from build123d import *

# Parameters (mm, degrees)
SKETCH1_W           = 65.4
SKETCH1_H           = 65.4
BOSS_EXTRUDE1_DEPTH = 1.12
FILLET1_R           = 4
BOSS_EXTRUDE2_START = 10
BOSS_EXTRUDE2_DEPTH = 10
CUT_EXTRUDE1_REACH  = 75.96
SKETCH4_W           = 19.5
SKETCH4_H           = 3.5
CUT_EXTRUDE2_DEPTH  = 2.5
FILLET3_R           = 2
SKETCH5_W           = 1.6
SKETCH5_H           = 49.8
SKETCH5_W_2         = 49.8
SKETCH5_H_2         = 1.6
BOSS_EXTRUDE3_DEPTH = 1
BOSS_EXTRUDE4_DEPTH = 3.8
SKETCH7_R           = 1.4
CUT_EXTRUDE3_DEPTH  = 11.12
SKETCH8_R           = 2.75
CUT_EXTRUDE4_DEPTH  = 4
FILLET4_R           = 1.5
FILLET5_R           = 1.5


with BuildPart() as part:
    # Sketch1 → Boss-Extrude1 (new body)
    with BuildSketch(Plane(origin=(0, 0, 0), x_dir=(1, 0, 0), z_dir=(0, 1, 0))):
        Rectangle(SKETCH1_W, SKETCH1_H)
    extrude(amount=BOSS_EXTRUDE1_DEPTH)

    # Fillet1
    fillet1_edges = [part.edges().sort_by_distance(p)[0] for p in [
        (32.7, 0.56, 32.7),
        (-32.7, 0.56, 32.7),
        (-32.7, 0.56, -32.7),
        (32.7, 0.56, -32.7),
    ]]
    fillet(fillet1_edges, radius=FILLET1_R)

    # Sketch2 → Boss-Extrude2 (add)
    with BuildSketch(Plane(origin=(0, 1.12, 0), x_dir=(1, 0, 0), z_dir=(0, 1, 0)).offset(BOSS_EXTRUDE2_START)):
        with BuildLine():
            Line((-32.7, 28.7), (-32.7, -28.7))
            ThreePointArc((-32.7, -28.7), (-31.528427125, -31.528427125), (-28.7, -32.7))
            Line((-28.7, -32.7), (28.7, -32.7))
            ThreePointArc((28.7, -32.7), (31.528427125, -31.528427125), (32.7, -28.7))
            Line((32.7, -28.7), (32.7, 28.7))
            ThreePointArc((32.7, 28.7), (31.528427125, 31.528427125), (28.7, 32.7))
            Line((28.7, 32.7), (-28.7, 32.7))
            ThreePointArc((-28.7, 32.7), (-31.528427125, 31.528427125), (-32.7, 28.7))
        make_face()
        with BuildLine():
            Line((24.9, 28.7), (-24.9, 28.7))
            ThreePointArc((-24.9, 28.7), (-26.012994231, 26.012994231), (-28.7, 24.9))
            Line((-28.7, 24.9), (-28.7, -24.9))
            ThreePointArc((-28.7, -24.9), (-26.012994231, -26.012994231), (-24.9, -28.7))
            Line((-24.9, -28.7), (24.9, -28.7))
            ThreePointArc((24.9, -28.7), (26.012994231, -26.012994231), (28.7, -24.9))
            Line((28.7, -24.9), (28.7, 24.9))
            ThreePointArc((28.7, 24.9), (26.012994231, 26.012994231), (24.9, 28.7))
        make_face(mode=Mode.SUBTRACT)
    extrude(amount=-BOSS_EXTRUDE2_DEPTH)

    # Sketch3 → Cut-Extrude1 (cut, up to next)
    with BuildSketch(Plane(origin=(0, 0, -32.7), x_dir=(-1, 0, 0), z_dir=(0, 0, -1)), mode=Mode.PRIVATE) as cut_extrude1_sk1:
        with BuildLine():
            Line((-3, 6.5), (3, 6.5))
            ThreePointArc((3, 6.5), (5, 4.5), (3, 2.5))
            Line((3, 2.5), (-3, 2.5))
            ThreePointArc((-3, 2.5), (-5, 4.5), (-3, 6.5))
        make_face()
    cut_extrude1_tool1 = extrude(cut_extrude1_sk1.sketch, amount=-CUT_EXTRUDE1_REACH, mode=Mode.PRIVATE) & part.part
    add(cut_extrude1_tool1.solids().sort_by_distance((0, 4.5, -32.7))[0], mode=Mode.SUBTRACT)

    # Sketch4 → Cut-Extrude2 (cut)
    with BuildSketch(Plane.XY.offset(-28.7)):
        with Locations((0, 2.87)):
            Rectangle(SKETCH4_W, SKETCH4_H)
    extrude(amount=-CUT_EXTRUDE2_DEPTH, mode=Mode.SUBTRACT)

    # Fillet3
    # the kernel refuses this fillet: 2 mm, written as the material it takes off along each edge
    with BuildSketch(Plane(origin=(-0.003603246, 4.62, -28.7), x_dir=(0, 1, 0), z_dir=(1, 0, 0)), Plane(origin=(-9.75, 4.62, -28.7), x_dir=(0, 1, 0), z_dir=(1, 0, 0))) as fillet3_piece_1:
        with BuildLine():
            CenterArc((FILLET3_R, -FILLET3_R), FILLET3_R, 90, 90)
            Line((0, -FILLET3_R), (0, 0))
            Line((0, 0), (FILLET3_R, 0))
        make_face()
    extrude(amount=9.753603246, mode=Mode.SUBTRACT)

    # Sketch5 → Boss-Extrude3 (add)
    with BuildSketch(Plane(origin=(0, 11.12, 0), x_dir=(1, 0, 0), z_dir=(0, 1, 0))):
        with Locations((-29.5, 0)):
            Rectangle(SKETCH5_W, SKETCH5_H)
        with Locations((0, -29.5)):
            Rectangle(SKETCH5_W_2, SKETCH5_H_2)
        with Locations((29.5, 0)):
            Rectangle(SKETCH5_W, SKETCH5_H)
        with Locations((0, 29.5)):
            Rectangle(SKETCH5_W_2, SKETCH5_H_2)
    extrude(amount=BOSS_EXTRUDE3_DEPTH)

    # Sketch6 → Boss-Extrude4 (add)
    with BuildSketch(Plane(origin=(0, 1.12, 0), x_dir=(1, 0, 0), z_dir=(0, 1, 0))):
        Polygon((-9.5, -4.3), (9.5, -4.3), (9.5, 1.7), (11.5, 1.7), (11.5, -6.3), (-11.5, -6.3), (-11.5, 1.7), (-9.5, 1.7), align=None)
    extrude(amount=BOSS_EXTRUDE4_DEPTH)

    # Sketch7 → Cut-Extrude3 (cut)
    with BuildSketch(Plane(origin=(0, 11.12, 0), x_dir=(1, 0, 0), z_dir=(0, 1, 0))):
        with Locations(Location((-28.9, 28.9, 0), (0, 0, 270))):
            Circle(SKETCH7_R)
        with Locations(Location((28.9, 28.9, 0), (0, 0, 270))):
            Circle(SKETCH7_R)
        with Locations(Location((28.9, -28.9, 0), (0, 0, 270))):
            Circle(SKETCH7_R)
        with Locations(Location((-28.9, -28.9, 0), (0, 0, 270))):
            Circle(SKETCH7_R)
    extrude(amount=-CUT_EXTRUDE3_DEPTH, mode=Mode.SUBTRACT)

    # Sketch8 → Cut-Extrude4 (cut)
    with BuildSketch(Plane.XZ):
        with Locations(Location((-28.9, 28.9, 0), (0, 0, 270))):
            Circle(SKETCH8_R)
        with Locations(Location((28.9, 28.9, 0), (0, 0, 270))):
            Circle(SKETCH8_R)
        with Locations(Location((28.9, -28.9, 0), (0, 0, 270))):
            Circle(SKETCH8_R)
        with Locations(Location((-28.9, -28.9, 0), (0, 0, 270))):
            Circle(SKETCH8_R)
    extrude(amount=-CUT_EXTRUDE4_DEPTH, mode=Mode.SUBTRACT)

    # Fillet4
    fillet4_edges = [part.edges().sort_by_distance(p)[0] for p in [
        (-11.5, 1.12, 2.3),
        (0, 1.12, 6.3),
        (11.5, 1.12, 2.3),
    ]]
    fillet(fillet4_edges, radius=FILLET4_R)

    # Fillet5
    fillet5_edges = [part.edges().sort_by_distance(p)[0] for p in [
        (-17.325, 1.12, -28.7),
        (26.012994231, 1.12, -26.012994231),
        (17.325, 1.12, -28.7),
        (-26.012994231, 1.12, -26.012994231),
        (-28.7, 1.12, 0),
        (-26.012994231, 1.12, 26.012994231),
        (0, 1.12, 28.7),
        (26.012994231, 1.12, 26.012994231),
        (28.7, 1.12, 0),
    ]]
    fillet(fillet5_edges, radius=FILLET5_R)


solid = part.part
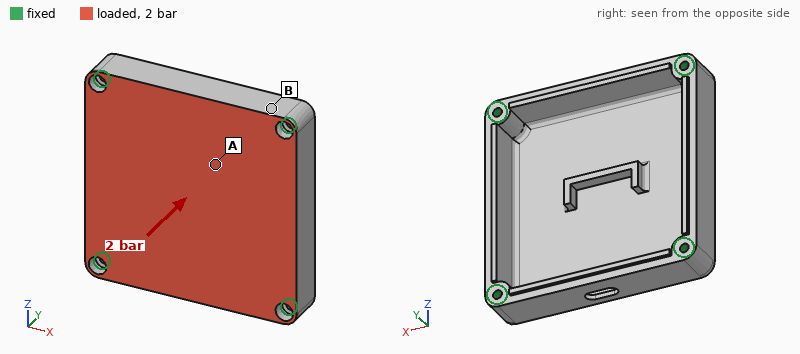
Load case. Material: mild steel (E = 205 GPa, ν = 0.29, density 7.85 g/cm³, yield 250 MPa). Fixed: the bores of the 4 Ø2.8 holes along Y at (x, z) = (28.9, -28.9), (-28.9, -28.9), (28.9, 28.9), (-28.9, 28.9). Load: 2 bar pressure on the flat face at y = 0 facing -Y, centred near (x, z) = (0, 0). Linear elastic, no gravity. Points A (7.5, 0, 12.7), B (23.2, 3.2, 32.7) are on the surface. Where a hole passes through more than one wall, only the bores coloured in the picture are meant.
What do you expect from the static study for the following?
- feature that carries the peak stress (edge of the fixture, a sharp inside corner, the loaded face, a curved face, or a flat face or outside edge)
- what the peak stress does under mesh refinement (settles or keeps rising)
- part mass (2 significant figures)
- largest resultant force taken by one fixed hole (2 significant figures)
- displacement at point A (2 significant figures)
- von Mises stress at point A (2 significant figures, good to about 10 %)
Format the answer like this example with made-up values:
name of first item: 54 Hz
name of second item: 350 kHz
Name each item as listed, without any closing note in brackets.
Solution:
feature that carries the peak stress: a sharp inside corner
what the peak stress does under mesh refinement: keeps rising
part mass: 120 g
largest resultant force taken by one fixed hole: 260 N
displacement at point A: 52 µm
von Mises stress at point A: 38 MPa
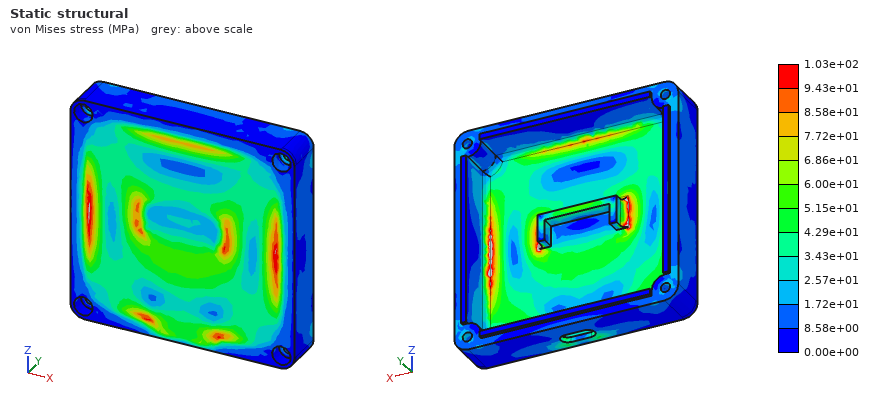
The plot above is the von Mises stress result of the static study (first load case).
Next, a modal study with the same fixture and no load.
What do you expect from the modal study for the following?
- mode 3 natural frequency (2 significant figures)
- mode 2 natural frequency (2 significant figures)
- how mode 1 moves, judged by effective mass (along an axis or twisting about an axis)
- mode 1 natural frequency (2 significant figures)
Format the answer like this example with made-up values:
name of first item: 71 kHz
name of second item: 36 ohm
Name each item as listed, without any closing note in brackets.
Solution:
mode 3 natural frequency: 5800 Hz
mode 2 natural frequency: 5500 Hz
how mode 1 moves, judged by effective mass: along Y
mode 1 natural frequency: 3000 Hz
